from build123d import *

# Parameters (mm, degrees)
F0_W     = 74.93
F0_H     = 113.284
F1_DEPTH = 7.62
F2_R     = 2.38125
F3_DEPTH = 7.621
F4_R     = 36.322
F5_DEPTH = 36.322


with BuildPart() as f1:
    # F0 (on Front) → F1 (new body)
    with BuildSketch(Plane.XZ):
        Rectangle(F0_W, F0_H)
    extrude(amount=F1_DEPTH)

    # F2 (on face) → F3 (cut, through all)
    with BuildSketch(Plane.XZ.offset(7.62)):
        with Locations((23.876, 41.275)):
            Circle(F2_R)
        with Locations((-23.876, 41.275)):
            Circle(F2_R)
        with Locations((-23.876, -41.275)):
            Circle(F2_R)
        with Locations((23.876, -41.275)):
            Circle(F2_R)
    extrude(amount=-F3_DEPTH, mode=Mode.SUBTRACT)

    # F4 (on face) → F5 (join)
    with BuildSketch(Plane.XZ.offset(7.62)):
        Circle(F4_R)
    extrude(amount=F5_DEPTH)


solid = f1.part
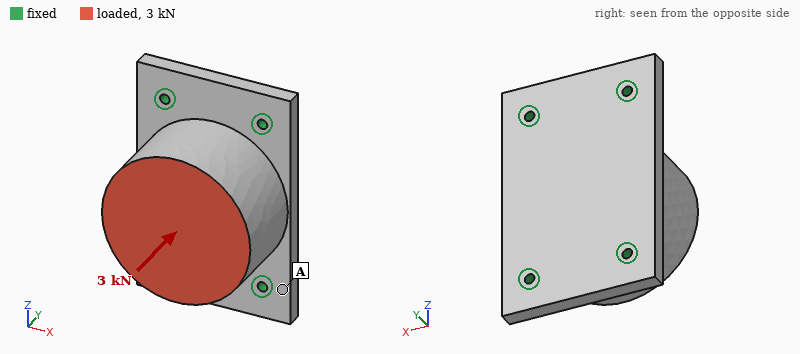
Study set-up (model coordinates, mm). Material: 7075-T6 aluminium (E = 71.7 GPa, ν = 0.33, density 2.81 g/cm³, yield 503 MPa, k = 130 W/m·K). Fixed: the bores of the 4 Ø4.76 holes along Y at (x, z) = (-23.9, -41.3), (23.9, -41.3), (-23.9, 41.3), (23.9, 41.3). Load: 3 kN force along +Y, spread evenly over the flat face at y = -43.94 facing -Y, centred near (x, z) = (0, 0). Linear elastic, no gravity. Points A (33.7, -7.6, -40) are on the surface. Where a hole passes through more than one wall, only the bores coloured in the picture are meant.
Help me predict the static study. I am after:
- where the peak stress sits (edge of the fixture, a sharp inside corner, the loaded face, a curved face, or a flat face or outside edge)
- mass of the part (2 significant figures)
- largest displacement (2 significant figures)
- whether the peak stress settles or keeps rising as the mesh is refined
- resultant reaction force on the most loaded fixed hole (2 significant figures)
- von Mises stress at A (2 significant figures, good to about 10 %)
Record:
edge of the fixture
600 g
7.2 µm
keeps rising
820 N
3.9 MPa
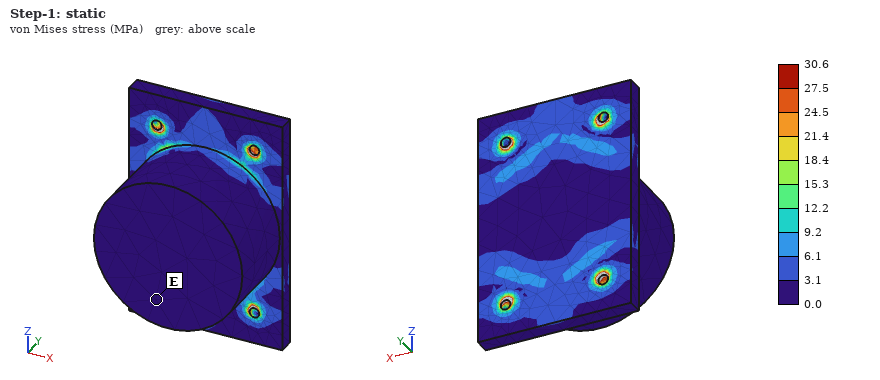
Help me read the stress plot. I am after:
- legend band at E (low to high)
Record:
0.0 to 3.1 MPa
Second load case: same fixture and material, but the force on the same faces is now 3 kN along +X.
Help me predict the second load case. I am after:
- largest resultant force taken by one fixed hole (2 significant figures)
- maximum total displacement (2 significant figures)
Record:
1.6 kN
32 µm
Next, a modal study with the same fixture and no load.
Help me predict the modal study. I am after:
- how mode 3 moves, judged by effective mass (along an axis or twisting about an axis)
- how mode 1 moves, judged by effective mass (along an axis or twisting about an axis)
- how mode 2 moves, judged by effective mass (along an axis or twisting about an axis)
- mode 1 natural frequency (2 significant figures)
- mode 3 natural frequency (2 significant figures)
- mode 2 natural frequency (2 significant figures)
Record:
along Z
along X
along Y
3500 Hz
5700 Hz
4600 Hz
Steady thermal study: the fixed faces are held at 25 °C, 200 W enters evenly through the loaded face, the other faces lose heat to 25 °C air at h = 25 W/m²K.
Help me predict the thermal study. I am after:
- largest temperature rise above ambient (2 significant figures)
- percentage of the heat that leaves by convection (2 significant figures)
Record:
44 K
7.1 %
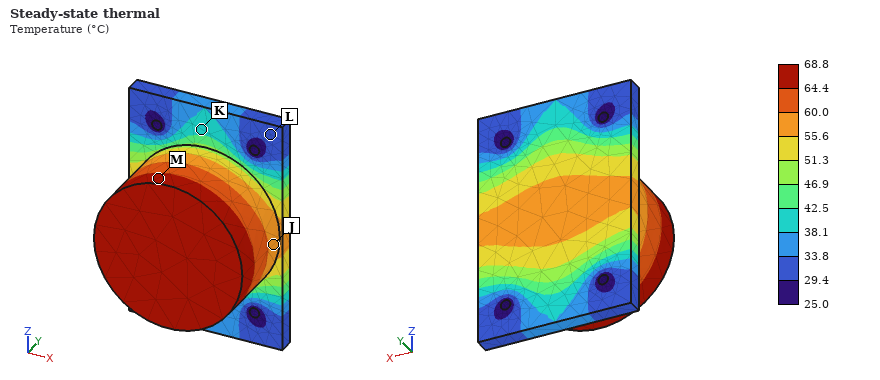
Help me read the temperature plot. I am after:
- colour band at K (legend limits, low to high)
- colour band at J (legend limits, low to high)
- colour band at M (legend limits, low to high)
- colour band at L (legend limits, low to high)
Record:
38.1 to 42.5 °C
55.6 to 60.0 °C
64.4 to 68.8 °C
29.4 to 33.8 °C
